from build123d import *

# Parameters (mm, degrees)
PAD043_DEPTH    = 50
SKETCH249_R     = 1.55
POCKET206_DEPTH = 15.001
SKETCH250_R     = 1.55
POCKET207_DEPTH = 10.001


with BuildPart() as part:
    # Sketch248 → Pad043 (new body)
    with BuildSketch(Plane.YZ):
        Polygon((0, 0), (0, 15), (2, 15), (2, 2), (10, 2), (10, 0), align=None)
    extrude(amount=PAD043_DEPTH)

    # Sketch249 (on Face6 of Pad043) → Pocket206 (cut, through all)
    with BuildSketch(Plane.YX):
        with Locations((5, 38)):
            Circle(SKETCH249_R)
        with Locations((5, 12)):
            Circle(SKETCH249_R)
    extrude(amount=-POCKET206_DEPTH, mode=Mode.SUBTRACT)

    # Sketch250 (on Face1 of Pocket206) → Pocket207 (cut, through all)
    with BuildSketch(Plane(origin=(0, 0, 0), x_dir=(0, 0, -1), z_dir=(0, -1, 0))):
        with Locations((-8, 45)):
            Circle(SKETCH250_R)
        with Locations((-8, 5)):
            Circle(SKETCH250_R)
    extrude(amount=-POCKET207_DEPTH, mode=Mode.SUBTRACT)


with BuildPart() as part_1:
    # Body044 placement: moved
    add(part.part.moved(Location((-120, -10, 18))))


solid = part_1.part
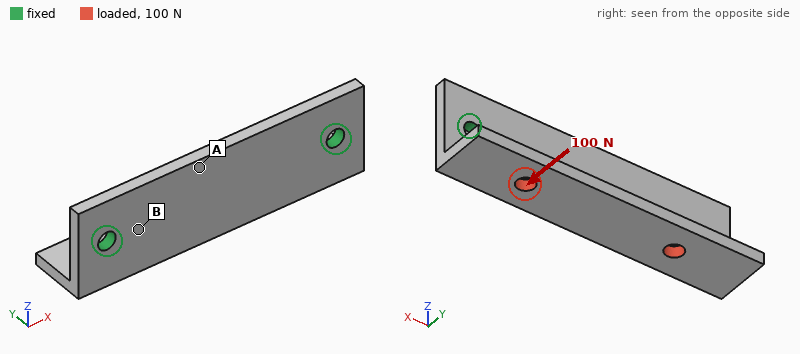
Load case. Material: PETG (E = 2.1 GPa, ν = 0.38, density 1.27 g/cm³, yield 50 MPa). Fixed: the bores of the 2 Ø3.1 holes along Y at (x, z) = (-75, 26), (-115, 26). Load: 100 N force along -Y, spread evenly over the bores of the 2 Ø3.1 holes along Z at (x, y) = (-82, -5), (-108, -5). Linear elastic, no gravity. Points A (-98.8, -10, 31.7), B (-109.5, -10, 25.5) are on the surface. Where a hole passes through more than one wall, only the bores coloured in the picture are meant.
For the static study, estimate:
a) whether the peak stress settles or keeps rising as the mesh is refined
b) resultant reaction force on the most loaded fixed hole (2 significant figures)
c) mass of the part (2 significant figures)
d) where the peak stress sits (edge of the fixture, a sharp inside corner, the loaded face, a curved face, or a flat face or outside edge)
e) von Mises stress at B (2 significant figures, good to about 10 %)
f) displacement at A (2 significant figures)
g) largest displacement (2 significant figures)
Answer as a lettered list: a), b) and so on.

a) keeps rising
b) 54 N
c) 2.8 g
d) edge of the fixture
e) 10.0 MPa
f) 0.11 mm
g) 0.59 mm
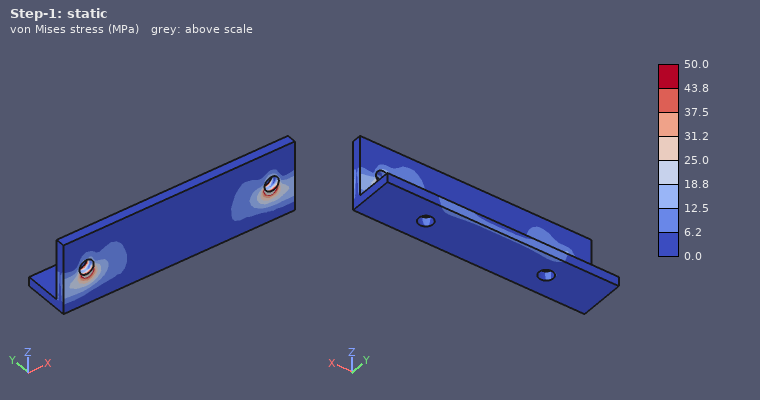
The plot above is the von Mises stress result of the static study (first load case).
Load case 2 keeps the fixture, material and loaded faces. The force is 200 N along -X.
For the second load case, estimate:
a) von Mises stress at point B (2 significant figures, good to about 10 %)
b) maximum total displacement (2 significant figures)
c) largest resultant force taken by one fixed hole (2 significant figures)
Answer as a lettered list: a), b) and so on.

a) 4.1 MPa
b) 0.20 mm
c) 110 N
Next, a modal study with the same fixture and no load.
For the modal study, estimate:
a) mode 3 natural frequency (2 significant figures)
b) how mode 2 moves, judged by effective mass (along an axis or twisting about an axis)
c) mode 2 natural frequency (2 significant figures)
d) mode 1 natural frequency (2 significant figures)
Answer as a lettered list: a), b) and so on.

a) 2800 Hz
b) along Y
c) 2300 Hz
d) 1700 Hz
